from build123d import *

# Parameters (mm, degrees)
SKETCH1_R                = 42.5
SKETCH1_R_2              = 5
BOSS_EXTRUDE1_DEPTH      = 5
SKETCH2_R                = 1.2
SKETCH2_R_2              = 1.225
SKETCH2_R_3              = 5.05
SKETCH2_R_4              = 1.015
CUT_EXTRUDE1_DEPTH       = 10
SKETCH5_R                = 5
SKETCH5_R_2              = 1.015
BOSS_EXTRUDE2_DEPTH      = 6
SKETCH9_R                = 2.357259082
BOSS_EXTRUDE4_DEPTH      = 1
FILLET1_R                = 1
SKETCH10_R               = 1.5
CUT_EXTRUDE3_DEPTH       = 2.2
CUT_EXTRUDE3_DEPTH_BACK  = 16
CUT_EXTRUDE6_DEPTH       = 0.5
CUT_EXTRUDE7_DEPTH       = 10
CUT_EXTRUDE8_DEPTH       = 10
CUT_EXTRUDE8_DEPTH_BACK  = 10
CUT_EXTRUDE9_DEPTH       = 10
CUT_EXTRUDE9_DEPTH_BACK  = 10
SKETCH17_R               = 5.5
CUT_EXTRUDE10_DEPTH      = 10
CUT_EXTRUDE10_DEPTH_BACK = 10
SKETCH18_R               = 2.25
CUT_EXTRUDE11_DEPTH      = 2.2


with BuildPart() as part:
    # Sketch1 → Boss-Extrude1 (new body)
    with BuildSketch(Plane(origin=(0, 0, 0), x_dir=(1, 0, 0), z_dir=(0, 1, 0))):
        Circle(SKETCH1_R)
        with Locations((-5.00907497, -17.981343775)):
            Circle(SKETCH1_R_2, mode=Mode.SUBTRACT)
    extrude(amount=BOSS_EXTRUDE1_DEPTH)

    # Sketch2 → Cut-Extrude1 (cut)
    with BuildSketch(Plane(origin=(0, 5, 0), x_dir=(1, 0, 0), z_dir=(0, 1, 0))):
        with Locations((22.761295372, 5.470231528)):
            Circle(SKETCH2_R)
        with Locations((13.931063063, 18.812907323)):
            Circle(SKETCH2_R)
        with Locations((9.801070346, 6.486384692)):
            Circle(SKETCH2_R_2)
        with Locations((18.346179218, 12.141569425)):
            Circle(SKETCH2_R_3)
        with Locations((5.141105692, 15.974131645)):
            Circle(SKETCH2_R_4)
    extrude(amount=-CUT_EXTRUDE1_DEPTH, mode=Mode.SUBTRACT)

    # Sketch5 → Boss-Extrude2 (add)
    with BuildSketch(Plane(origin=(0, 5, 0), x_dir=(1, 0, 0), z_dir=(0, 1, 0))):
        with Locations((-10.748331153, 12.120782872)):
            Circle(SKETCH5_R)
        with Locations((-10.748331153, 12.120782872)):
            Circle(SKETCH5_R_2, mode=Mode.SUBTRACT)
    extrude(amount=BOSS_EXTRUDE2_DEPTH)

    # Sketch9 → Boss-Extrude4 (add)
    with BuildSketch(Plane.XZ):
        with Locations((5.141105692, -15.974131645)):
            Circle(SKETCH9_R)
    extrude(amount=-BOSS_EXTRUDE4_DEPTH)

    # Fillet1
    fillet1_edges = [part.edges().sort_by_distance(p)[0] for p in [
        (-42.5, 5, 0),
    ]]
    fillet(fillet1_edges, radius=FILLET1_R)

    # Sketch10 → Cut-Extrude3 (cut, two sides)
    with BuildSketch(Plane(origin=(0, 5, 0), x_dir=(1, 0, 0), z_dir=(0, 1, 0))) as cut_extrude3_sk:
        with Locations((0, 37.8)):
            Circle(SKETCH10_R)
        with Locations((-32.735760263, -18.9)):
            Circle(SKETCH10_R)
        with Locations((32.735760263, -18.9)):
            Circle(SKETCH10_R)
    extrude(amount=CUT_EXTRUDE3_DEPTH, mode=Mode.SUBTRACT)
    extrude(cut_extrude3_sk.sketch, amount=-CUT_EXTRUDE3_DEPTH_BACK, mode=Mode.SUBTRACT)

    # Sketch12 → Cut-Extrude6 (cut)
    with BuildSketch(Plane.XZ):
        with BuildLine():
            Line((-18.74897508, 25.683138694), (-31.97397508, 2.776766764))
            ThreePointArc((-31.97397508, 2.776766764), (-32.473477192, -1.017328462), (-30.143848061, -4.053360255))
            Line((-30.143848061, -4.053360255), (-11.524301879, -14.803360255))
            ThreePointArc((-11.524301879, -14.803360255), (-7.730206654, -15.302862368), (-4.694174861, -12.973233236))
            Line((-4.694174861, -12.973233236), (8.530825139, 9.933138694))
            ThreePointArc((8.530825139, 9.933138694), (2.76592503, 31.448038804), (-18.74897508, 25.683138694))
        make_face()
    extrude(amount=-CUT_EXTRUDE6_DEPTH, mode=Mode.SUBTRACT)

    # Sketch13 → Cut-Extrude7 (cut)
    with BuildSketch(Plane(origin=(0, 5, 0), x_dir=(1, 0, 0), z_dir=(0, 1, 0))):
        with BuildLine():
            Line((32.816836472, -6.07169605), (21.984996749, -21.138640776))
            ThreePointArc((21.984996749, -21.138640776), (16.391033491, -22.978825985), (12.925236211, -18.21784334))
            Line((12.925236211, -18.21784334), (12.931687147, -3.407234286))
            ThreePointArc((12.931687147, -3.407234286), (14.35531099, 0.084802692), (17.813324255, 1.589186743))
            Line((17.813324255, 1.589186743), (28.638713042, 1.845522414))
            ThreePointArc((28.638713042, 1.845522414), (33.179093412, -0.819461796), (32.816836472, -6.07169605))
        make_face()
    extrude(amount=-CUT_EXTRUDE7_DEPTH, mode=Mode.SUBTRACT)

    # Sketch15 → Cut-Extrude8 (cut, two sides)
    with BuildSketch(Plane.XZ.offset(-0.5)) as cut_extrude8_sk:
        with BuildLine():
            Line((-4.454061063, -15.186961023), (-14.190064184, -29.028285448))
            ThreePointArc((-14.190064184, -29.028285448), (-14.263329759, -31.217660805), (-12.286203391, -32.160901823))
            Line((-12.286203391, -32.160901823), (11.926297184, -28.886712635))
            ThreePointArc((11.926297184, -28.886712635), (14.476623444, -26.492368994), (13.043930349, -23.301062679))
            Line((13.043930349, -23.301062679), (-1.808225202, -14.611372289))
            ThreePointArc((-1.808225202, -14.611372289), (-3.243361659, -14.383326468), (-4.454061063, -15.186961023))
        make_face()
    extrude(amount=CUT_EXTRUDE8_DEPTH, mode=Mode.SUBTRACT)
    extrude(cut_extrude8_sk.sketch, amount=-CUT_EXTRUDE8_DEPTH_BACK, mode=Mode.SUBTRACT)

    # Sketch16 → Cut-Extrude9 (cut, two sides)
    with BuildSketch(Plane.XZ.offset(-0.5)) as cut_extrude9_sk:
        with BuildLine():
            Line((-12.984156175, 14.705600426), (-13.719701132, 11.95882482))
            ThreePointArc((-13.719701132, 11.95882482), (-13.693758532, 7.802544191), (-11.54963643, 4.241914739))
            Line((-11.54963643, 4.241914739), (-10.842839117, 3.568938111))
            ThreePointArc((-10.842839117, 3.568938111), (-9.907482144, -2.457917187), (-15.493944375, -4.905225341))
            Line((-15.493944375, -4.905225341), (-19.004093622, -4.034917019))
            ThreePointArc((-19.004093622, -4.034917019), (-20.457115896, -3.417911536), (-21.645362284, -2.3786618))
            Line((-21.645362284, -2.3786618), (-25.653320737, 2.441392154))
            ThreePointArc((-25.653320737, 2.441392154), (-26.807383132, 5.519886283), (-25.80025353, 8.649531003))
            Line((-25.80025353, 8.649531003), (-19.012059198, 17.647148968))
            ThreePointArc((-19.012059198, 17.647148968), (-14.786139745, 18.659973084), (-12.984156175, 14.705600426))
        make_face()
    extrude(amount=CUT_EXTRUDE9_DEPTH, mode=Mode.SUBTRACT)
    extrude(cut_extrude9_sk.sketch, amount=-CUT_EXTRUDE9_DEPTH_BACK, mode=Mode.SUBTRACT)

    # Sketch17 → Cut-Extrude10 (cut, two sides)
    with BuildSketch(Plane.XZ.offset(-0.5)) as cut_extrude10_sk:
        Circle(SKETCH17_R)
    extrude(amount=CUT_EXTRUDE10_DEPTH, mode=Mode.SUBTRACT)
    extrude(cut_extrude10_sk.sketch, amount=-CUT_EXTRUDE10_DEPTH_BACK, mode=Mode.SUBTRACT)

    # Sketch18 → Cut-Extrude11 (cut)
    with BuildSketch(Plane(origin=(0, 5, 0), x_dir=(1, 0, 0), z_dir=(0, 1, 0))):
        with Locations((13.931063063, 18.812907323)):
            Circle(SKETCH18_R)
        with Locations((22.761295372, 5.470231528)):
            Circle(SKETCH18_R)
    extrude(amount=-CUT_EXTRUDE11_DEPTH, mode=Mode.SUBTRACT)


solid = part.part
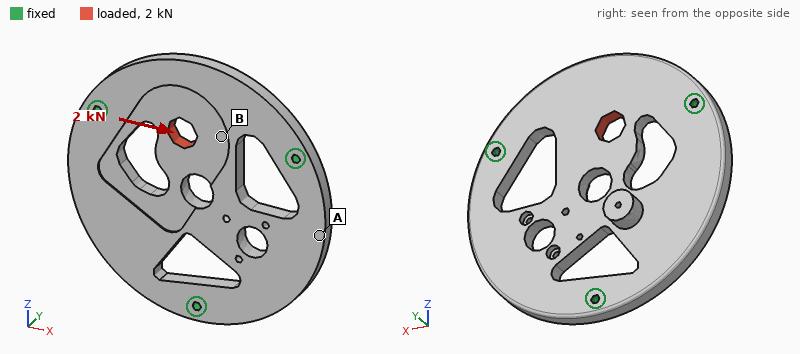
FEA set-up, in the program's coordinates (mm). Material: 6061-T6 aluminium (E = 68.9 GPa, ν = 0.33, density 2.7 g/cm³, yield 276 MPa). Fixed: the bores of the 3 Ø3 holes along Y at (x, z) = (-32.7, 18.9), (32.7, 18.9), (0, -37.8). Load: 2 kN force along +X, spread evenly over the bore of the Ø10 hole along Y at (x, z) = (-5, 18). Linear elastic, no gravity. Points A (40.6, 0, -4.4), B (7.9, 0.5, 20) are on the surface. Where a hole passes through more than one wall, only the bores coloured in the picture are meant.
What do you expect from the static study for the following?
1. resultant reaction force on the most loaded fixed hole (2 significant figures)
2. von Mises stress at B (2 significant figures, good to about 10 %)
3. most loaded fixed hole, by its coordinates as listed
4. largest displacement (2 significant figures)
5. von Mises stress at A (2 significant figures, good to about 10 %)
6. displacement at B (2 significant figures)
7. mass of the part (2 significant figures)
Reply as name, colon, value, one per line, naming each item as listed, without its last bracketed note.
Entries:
resultant reaction force on the most loaded fixed hole: 1.1 kN
von Mises stress at B: 16 MPa
most loaded fixed hole, by its coordinates as listed: (-32.7, 18.9)
largest displacement: 15 µm
von Mises stress at A: 6.3 MPa
displacement at B: 11 µm
mass of the part: 60 g
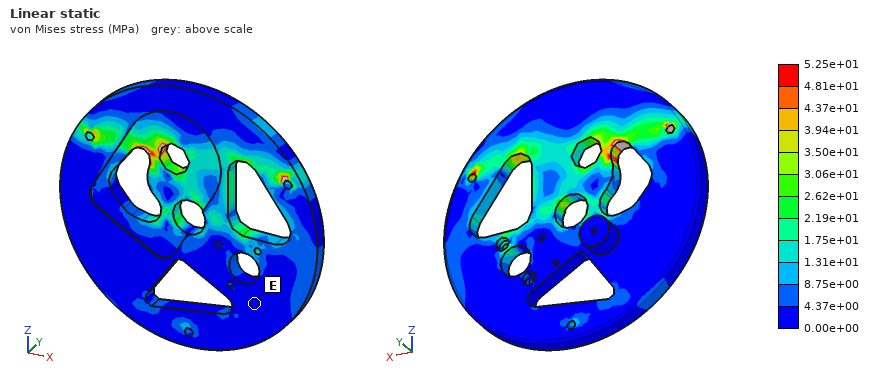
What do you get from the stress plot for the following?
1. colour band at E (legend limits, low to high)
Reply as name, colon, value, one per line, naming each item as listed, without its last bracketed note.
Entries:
colour band at E: 0.00e+00 to 4.37e+00 MPa
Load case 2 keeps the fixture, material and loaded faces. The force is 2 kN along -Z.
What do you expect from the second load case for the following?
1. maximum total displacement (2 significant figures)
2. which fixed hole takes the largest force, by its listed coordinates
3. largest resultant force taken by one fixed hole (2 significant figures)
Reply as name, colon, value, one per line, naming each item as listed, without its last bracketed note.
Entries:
maximum total displacement: 14 µm
which fixed hole takes the largest force, by its listed coordinates: (-32.7, 18.9)
largest resultant force taken by one fixed hole: 1.2 kN
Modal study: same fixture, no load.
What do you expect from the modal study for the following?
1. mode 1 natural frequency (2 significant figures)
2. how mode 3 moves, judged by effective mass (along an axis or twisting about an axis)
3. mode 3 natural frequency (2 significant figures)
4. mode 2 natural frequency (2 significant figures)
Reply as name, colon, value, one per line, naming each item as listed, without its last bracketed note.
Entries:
mode 1 natural frequency: 3600 Hz
how mode 3 moves, judged by effective mass: along Y
mode 3 natural frequency: 3800 Hz
mode 2 natural frequency: 3600 Hz
